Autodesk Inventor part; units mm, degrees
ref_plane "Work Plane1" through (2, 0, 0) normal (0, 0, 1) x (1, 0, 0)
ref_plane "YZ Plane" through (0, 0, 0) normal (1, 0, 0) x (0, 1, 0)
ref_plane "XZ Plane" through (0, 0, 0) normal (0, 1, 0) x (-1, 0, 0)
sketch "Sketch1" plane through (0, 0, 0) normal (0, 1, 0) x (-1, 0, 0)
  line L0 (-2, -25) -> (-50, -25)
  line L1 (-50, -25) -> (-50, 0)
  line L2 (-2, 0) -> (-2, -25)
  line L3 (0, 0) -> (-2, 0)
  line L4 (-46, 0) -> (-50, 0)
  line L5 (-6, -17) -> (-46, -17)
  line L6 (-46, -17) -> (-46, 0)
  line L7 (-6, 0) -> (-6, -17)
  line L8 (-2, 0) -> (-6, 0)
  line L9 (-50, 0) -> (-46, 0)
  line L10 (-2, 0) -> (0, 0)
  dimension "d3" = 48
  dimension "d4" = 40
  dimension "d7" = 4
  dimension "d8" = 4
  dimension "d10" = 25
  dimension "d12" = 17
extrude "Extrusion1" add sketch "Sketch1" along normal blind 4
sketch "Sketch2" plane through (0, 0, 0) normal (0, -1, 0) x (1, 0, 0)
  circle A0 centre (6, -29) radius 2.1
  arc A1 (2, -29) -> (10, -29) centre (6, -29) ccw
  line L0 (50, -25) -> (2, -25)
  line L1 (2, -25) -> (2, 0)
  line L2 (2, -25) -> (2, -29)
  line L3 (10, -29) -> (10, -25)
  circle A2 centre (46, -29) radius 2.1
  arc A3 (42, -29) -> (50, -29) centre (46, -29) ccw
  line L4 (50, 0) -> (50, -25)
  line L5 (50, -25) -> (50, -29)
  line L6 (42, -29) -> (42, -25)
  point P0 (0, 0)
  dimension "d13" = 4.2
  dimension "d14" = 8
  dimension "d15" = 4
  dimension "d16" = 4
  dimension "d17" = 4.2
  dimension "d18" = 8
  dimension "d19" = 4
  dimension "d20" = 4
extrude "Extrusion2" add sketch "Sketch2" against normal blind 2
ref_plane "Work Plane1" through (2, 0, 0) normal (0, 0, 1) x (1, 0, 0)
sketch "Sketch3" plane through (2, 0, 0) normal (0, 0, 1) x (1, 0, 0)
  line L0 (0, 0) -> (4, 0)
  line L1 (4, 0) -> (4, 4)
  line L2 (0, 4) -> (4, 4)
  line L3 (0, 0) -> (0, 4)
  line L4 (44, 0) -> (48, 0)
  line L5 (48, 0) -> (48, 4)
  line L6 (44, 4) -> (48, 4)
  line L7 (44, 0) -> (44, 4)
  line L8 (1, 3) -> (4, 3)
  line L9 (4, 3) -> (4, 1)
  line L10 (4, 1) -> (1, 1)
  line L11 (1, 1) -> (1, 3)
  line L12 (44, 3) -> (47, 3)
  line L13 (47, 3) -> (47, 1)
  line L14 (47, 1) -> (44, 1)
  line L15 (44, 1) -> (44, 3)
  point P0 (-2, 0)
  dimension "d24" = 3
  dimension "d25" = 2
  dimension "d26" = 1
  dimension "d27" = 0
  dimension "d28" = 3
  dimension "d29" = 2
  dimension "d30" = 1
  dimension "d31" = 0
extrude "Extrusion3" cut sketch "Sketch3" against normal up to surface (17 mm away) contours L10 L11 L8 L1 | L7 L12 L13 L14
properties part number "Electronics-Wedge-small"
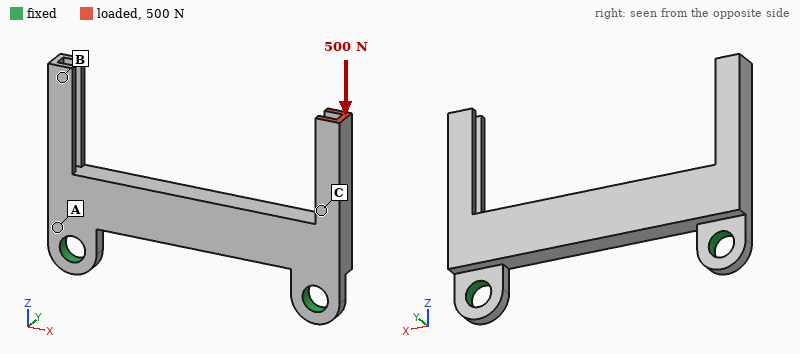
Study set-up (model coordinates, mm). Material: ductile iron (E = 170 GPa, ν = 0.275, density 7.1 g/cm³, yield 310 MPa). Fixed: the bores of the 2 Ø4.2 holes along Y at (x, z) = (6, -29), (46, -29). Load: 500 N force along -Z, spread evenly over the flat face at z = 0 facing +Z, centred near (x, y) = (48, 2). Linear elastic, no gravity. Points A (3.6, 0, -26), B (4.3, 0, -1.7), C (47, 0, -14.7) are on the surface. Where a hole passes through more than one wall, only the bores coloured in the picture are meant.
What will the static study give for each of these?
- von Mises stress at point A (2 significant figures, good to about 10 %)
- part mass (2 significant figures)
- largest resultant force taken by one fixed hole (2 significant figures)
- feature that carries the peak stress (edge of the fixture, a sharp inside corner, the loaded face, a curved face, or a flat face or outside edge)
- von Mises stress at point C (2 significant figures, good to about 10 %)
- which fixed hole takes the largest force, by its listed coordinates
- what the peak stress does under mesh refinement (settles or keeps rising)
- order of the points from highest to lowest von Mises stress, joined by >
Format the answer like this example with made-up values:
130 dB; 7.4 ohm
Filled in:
21 MPa; 15 g; 520 N; edge of the fixture; 48 MPa; (46, -29); keeps rising; C > A > B
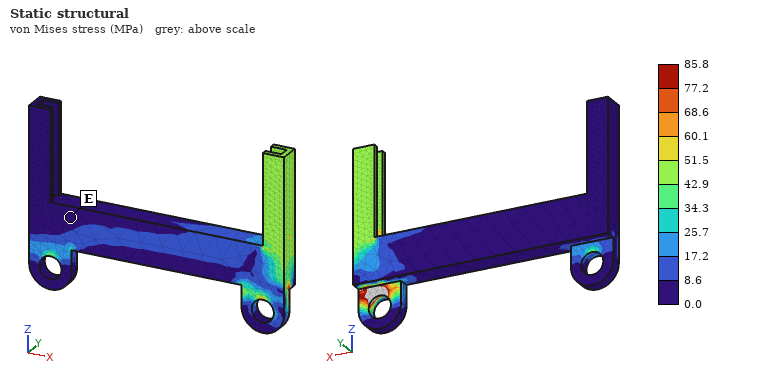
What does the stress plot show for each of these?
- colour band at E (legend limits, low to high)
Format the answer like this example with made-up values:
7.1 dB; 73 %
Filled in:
0.0 to 8.6 MPa
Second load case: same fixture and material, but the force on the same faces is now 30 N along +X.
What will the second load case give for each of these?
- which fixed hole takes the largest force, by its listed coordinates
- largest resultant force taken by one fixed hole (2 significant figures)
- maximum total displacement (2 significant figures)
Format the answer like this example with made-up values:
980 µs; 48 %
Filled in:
(6, -29); 42 N; 32 µm
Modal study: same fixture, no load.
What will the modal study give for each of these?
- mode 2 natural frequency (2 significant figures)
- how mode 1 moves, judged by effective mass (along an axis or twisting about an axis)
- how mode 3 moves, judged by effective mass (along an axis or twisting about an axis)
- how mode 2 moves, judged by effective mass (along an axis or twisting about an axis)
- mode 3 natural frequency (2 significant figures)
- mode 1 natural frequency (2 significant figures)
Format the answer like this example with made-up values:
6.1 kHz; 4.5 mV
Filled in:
4600 Hz; along Y; along Y; twisting about Z; 7200 Hz; 3200 Hz
